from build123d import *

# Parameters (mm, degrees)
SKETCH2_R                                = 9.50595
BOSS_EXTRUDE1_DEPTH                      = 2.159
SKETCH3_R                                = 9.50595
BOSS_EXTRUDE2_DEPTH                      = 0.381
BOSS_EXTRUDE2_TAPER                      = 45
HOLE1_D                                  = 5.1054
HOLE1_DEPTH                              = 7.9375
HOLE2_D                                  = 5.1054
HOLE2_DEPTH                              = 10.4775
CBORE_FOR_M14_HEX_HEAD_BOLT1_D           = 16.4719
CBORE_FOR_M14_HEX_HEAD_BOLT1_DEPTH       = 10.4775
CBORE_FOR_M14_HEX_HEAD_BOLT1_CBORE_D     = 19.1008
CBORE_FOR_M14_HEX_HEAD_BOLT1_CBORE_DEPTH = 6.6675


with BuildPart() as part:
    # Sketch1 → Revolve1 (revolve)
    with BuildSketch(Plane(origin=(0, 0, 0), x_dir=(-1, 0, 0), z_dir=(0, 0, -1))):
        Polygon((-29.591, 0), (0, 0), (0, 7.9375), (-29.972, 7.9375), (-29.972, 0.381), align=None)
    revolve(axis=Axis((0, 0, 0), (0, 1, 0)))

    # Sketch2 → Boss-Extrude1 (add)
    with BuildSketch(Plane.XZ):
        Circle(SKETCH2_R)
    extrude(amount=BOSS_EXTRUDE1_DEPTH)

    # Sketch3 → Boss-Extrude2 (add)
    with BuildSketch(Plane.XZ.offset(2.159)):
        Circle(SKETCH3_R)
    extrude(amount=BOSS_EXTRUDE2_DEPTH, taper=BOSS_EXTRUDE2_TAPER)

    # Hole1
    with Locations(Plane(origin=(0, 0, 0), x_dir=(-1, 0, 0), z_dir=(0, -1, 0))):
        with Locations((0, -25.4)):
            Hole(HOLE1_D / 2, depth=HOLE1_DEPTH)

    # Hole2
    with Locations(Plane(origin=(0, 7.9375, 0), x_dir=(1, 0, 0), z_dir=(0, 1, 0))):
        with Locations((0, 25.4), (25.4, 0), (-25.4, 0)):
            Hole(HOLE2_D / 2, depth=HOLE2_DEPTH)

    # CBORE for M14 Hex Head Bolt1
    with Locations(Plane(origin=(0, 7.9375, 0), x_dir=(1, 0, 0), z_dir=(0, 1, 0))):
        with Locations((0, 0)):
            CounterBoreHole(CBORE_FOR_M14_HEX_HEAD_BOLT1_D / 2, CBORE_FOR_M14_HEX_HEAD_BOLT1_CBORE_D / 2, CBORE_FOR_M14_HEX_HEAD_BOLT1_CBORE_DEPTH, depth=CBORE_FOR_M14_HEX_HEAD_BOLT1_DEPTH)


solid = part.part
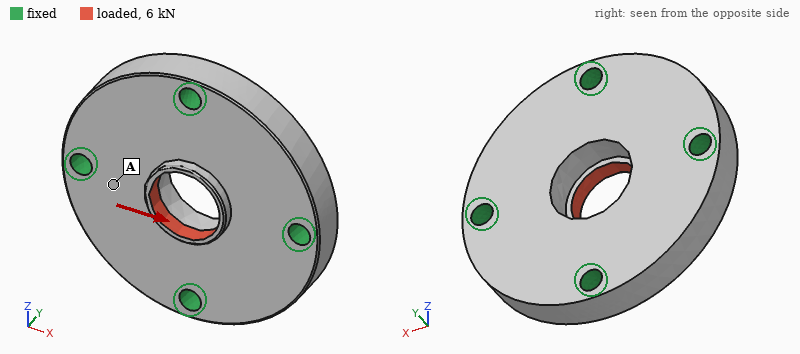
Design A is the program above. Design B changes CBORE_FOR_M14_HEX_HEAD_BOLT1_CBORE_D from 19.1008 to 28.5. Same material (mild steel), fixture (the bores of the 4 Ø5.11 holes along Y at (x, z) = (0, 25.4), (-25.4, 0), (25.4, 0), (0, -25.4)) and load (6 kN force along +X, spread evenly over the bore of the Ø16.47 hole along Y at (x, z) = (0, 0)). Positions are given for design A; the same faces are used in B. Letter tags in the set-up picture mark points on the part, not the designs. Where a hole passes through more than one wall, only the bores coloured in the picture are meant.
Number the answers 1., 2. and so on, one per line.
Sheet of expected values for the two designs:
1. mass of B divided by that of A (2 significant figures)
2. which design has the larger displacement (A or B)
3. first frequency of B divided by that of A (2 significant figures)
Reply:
1. 0.88
2. B
3. 1.0
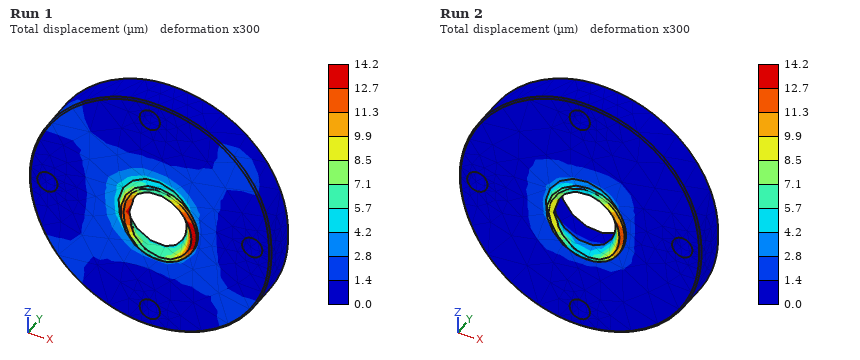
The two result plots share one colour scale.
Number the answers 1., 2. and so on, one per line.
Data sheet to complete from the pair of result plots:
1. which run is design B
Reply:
1. Run 1
